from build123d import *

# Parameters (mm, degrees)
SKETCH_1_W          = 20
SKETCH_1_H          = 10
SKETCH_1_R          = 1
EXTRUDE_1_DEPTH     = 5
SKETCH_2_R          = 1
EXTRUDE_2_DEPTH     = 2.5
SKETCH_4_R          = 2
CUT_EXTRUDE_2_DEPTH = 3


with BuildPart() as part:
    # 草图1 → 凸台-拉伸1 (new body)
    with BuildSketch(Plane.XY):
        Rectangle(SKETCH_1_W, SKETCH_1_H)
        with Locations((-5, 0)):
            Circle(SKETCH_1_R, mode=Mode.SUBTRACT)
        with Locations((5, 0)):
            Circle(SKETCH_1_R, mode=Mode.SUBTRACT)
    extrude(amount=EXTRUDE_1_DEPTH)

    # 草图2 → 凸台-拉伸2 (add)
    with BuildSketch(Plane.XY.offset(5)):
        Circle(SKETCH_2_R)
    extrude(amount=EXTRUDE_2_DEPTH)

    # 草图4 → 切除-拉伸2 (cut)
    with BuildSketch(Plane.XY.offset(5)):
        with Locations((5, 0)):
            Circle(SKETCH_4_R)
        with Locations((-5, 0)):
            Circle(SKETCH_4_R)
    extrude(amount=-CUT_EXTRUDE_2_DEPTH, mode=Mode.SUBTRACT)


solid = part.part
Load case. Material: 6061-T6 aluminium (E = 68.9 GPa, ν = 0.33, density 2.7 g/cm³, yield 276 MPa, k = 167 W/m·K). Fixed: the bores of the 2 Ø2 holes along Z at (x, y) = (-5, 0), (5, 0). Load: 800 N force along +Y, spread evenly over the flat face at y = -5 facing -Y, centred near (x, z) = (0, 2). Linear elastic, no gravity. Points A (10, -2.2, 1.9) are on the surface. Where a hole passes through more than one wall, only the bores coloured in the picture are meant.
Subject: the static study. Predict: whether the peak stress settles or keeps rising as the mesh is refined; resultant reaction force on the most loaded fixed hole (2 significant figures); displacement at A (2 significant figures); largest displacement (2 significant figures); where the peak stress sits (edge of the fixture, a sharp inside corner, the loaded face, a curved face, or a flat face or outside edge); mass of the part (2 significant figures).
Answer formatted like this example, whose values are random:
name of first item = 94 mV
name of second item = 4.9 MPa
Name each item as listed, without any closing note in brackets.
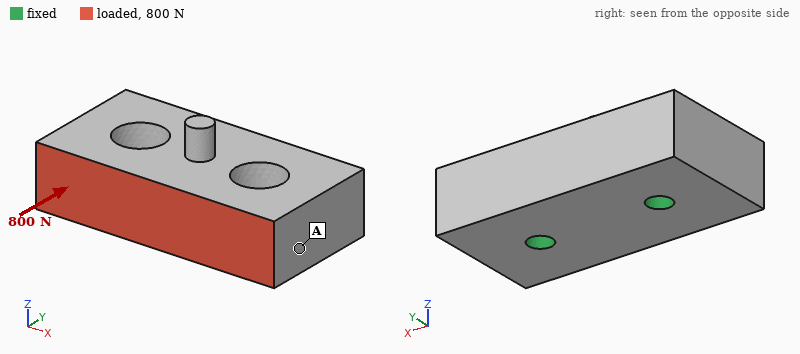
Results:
whether the peak stress settles or keeps rising as the mesh is refined = keeps rising
resultant reaction force on the most loaded fixed hole = 400 N
displacement at A = 3.8 µm
largest displacement = 9.7 µm
where the peak stress sits = edge of the fixture
mass of the part = 2.5 g
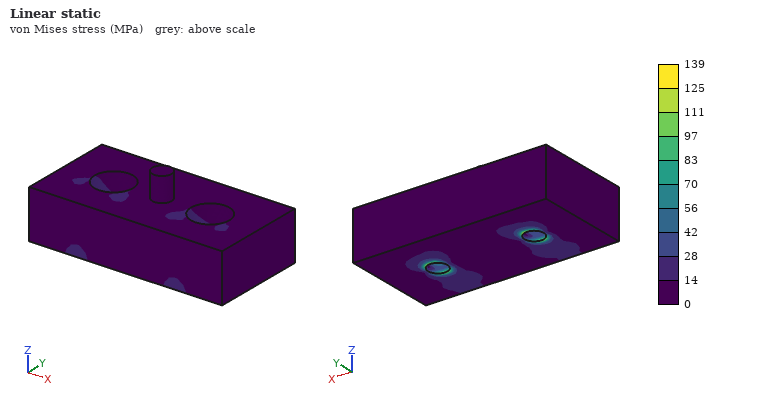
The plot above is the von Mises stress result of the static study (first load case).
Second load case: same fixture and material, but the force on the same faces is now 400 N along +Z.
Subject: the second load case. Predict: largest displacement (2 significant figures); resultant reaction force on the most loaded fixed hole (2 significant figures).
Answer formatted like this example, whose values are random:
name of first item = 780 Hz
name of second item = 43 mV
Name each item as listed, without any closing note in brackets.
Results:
largest displacement = 15 µm
resultant reaction force on the most loaded fixed hole = 200 N
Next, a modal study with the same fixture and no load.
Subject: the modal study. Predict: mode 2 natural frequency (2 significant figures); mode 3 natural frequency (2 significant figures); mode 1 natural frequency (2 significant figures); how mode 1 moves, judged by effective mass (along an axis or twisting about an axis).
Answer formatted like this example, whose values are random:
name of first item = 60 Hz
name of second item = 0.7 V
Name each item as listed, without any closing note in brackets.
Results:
mode 2 natural frequency = 49 kHz
mode 3 natural frequency = 50 kHz
mode 1 natural frequency = 28 kHz
how mode 1 moves, judged by effective mass = along Y
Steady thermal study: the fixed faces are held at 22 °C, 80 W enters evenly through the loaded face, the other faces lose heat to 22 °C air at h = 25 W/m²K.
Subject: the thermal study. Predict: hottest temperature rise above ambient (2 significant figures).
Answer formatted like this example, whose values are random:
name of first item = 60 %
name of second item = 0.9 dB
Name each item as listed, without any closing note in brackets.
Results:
hottest temperature rise above ambient = 43 K
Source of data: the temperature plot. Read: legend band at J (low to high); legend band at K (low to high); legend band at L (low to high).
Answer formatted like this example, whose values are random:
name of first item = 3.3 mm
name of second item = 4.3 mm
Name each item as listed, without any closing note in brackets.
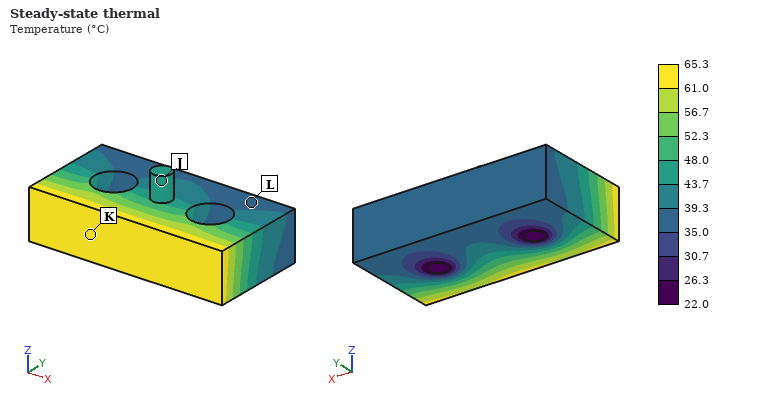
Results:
legend band at J = 43.7 to 48.0 °C
legend band at K = 61.0 to 65.3 °C
legend band at L = 35.0 to 39.3 °C
